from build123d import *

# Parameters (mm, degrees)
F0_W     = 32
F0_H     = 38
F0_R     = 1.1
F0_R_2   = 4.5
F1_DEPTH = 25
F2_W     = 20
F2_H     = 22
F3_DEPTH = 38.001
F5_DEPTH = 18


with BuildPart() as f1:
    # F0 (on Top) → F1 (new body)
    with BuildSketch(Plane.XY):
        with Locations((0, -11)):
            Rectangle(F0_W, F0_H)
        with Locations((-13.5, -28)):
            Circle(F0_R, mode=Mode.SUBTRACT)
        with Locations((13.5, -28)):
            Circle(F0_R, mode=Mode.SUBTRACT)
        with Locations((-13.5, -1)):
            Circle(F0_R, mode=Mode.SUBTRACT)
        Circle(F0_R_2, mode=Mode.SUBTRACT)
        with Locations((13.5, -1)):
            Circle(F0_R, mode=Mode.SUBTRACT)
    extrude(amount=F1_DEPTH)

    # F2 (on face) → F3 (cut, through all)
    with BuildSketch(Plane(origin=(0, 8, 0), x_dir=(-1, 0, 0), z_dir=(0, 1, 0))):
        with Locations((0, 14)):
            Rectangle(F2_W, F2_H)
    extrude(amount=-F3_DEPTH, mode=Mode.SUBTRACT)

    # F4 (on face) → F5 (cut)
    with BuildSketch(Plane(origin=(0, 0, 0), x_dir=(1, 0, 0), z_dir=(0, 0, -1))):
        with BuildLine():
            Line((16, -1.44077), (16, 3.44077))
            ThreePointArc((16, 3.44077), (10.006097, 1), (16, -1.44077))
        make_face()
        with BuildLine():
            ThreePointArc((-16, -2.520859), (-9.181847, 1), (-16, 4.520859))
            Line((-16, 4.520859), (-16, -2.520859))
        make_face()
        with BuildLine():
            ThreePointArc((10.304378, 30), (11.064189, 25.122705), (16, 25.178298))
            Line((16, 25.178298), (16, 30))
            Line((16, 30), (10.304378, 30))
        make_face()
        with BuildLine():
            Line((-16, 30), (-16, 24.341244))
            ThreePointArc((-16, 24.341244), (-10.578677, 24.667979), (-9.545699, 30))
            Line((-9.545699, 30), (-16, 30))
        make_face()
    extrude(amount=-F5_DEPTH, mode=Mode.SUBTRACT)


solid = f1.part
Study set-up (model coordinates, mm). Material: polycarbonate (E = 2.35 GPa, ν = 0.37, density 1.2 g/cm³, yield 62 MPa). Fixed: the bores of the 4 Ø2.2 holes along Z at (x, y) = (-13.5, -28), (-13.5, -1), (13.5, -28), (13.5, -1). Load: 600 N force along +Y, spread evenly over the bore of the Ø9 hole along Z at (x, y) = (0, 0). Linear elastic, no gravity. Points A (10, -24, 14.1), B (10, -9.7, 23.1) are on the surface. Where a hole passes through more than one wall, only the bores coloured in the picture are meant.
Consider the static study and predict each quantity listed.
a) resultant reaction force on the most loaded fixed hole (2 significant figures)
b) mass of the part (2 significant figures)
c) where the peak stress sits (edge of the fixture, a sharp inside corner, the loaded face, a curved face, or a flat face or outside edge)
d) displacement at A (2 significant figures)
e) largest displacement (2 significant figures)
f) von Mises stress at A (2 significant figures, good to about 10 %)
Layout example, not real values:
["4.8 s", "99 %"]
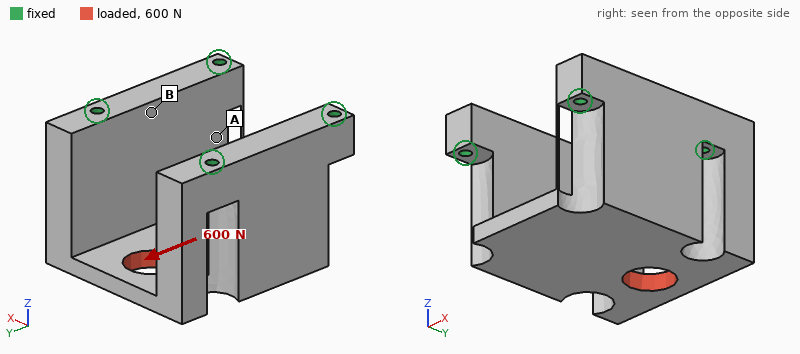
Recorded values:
["290 N", "13 g", "a flat face or outside edge", "0.060 mm", "0.30 mm", "9.5 MPa"]
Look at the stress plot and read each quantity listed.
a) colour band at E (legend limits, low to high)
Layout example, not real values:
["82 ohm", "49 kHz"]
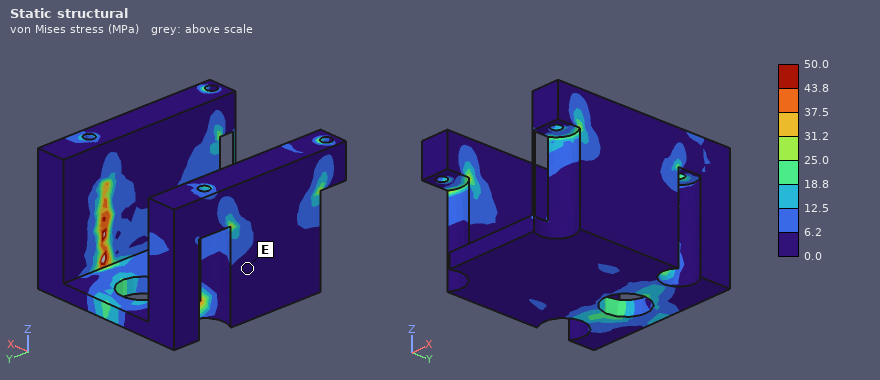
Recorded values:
["0.0 to 6.2 MPa"]
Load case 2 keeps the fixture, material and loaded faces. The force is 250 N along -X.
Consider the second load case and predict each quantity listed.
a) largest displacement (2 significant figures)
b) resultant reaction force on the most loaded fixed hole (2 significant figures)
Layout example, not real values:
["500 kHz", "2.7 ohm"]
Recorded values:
["0.48 mm", "100 N"]
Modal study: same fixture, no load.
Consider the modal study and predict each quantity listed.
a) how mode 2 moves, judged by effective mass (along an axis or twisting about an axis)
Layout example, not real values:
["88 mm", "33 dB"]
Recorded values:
["along X"]
